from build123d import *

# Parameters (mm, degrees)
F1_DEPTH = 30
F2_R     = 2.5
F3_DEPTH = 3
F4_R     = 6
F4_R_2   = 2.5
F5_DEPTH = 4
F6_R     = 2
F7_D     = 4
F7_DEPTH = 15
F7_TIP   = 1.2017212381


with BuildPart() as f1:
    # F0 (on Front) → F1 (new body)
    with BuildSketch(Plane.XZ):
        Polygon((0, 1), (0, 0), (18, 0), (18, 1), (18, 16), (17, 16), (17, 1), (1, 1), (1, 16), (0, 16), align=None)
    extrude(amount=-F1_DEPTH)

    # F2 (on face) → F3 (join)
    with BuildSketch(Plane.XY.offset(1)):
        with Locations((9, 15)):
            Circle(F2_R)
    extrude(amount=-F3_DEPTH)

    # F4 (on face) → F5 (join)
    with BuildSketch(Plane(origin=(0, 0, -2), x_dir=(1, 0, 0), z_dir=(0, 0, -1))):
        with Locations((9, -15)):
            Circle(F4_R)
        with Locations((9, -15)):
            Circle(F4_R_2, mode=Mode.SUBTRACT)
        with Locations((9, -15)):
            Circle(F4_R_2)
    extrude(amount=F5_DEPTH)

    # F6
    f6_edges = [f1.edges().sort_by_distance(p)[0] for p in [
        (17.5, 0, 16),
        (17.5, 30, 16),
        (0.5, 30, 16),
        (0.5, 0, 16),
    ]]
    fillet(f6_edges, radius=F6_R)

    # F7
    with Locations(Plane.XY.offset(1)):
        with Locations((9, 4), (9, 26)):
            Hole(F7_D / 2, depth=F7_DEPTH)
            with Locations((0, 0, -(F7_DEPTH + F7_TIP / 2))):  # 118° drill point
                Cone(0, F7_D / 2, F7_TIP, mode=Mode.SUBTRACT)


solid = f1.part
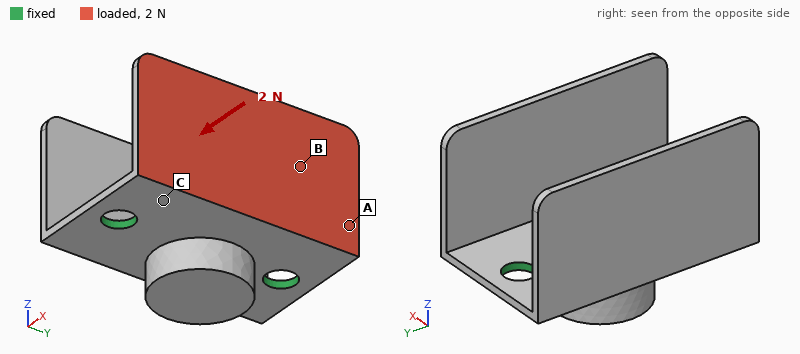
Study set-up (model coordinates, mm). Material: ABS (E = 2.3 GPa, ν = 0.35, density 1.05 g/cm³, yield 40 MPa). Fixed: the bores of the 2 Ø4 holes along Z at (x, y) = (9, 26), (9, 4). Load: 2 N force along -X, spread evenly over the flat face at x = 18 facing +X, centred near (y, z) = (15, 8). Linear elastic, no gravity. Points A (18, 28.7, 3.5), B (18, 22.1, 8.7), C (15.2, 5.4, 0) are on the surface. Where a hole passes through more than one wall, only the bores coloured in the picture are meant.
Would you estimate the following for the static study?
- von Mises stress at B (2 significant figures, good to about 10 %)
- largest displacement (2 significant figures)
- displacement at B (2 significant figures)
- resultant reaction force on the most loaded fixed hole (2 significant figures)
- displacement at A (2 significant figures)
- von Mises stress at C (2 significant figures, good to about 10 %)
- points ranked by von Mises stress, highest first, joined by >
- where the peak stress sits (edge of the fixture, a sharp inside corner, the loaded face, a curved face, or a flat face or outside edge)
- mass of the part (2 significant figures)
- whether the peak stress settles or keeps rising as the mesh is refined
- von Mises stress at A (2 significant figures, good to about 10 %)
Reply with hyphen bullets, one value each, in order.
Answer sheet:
- 0.58 MPa
- 0.40 mm
- 0.21 mm
- 1.0 N
- 0.096 mm
- 2.5 MPa
- C > A > B
- edge of the fixture
- 2.0 g
- keeps rising
- 1.7 MPa
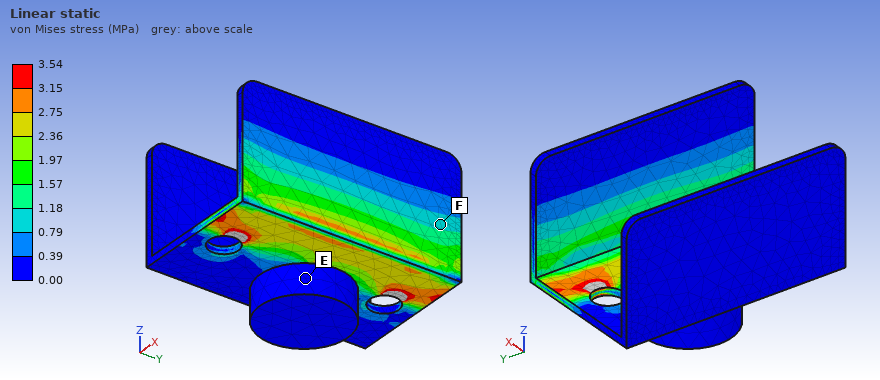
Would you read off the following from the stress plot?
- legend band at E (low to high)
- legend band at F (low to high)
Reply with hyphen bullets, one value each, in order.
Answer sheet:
- 0.00 to 0.39 MPa
- 0.79 to 1.18 MPa
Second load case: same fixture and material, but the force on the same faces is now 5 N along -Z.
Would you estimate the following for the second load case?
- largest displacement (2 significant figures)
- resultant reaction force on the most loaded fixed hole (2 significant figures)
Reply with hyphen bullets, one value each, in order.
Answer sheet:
- 0.44 mm
- 2.5 N
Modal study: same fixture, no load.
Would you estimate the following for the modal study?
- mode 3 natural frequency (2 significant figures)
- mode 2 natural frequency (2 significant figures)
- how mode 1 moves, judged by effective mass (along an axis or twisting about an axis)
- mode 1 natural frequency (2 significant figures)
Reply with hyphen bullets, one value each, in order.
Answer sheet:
- 1100 Hz
- 610 Hz
- along X
- 580 Hz
